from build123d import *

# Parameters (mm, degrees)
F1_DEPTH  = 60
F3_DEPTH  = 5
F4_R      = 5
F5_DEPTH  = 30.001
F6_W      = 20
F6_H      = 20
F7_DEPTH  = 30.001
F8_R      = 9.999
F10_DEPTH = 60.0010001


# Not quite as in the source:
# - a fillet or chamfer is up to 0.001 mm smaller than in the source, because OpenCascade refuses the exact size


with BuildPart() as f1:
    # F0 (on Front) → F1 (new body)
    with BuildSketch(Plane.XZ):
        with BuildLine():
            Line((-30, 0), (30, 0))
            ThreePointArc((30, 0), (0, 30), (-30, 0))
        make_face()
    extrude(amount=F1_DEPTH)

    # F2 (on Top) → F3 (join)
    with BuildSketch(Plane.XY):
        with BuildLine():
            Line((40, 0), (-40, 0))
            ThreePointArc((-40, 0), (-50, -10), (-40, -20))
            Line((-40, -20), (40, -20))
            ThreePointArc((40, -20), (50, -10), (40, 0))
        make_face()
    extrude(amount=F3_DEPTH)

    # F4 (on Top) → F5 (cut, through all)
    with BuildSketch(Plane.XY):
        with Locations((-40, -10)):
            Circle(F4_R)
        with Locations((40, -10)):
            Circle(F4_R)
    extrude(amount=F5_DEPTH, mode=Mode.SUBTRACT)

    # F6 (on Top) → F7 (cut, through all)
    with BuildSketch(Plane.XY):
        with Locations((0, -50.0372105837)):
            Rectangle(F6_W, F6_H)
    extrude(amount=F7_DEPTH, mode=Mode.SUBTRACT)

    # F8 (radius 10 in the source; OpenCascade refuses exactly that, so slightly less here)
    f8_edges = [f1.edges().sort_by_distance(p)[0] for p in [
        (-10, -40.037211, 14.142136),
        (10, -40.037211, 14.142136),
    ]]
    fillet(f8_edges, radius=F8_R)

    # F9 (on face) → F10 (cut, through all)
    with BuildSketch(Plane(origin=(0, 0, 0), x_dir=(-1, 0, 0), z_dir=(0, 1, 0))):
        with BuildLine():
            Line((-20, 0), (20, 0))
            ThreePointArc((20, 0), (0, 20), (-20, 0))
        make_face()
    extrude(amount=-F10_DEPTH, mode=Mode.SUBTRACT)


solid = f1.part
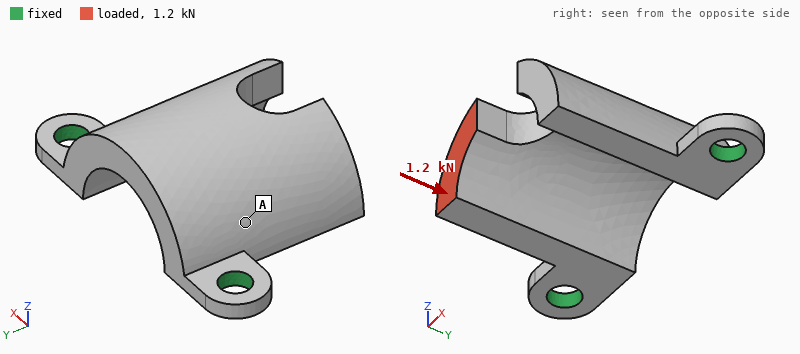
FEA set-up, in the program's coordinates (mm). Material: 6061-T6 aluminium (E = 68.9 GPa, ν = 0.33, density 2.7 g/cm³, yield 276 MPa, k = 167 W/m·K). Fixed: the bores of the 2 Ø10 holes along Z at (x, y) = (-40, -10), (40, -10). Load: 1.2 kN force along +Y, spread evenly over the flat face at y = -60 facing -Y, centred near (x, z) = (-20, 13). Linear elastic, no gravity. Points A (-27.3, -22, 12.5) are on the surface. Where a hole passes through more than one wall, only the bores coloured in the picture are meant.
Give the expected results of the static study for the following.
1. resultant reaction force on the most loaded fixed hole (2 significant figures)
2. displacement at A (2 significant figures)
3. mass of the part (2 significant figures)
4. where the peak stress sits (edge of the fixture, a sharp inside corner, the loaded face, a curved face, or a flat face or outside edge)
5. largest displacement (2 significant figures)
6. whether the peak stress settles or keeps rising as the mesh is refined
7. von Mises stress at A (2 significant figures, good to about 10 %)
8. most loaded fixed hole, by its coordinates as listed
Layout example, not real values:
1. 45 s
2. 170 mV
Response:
1. 970 N
2. 0.034 mm
3. 120 g
4. edge of the fixture
5. 0.11 mm
6. keeps rising
7. 11 MPa
8. (-40, -10)
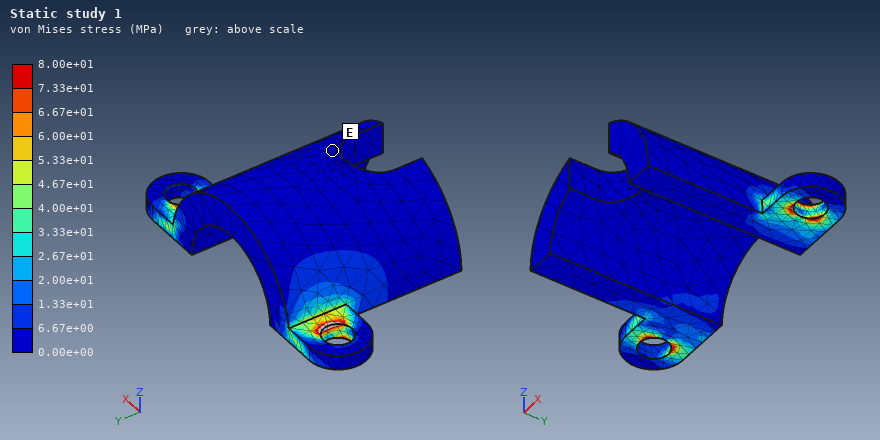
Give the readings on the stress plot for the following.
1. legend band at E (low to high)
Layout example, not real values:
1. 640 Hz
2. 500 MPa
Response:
1. 0.00e+00 to 6.67e+00 MPa
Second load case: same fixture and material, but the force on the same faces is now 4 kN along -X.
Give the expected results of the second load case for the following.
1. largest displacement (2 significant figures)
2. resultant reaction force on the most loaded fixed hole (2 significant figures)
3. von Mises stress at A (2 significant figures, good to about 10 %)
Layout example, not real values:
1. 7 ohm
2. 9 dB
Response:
1. 0.43 mm
2. 3.5 kN
3. 92 MPa
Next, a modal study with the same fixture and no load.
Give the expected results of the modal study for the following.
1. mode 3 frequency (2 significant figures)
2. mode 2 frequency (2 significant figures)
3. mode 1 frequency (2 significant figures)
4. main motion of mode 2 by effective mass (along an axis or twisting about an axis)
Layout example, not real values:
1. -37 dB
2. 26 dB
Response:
1. 6100 Hz
2. 3600 Hz
3. 1300 Hz
4. along X
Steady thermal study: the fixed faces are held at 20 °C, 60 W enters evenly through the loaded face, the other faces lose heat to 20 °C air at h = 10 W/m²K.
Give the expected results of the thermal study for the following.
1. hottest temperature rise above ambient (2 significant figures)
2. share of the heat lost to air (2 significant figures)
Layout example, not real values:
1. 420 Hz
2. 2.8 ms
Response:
1. 70 K
2. 5.6 %
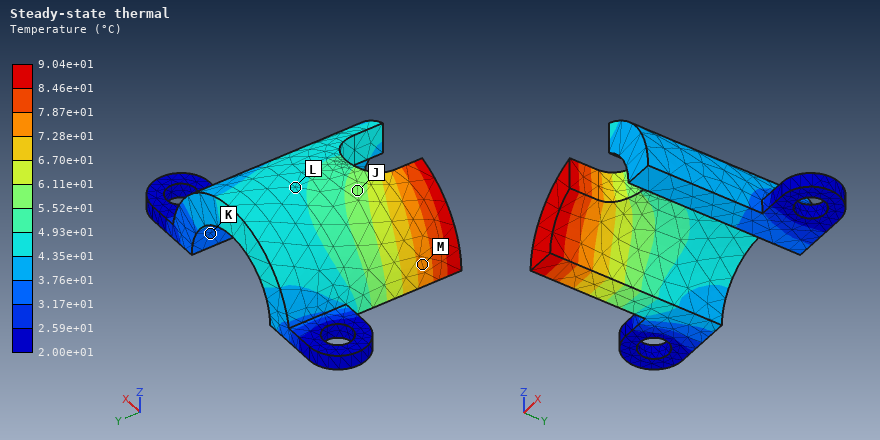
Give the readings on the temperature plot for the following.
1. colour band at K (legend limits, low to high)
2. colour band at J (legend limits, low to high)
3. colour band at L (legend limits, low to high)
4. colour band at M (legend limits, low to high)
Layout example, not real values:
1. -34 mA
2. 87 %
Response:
1. 3.17e+01 to 3.76e+01 °C
2. 5.52e+01 to 6.11e+01 °C
3. 4.35e+01 to 4.93e+01 °C
4. 7.28e+01 to 7.87e+01 °C
